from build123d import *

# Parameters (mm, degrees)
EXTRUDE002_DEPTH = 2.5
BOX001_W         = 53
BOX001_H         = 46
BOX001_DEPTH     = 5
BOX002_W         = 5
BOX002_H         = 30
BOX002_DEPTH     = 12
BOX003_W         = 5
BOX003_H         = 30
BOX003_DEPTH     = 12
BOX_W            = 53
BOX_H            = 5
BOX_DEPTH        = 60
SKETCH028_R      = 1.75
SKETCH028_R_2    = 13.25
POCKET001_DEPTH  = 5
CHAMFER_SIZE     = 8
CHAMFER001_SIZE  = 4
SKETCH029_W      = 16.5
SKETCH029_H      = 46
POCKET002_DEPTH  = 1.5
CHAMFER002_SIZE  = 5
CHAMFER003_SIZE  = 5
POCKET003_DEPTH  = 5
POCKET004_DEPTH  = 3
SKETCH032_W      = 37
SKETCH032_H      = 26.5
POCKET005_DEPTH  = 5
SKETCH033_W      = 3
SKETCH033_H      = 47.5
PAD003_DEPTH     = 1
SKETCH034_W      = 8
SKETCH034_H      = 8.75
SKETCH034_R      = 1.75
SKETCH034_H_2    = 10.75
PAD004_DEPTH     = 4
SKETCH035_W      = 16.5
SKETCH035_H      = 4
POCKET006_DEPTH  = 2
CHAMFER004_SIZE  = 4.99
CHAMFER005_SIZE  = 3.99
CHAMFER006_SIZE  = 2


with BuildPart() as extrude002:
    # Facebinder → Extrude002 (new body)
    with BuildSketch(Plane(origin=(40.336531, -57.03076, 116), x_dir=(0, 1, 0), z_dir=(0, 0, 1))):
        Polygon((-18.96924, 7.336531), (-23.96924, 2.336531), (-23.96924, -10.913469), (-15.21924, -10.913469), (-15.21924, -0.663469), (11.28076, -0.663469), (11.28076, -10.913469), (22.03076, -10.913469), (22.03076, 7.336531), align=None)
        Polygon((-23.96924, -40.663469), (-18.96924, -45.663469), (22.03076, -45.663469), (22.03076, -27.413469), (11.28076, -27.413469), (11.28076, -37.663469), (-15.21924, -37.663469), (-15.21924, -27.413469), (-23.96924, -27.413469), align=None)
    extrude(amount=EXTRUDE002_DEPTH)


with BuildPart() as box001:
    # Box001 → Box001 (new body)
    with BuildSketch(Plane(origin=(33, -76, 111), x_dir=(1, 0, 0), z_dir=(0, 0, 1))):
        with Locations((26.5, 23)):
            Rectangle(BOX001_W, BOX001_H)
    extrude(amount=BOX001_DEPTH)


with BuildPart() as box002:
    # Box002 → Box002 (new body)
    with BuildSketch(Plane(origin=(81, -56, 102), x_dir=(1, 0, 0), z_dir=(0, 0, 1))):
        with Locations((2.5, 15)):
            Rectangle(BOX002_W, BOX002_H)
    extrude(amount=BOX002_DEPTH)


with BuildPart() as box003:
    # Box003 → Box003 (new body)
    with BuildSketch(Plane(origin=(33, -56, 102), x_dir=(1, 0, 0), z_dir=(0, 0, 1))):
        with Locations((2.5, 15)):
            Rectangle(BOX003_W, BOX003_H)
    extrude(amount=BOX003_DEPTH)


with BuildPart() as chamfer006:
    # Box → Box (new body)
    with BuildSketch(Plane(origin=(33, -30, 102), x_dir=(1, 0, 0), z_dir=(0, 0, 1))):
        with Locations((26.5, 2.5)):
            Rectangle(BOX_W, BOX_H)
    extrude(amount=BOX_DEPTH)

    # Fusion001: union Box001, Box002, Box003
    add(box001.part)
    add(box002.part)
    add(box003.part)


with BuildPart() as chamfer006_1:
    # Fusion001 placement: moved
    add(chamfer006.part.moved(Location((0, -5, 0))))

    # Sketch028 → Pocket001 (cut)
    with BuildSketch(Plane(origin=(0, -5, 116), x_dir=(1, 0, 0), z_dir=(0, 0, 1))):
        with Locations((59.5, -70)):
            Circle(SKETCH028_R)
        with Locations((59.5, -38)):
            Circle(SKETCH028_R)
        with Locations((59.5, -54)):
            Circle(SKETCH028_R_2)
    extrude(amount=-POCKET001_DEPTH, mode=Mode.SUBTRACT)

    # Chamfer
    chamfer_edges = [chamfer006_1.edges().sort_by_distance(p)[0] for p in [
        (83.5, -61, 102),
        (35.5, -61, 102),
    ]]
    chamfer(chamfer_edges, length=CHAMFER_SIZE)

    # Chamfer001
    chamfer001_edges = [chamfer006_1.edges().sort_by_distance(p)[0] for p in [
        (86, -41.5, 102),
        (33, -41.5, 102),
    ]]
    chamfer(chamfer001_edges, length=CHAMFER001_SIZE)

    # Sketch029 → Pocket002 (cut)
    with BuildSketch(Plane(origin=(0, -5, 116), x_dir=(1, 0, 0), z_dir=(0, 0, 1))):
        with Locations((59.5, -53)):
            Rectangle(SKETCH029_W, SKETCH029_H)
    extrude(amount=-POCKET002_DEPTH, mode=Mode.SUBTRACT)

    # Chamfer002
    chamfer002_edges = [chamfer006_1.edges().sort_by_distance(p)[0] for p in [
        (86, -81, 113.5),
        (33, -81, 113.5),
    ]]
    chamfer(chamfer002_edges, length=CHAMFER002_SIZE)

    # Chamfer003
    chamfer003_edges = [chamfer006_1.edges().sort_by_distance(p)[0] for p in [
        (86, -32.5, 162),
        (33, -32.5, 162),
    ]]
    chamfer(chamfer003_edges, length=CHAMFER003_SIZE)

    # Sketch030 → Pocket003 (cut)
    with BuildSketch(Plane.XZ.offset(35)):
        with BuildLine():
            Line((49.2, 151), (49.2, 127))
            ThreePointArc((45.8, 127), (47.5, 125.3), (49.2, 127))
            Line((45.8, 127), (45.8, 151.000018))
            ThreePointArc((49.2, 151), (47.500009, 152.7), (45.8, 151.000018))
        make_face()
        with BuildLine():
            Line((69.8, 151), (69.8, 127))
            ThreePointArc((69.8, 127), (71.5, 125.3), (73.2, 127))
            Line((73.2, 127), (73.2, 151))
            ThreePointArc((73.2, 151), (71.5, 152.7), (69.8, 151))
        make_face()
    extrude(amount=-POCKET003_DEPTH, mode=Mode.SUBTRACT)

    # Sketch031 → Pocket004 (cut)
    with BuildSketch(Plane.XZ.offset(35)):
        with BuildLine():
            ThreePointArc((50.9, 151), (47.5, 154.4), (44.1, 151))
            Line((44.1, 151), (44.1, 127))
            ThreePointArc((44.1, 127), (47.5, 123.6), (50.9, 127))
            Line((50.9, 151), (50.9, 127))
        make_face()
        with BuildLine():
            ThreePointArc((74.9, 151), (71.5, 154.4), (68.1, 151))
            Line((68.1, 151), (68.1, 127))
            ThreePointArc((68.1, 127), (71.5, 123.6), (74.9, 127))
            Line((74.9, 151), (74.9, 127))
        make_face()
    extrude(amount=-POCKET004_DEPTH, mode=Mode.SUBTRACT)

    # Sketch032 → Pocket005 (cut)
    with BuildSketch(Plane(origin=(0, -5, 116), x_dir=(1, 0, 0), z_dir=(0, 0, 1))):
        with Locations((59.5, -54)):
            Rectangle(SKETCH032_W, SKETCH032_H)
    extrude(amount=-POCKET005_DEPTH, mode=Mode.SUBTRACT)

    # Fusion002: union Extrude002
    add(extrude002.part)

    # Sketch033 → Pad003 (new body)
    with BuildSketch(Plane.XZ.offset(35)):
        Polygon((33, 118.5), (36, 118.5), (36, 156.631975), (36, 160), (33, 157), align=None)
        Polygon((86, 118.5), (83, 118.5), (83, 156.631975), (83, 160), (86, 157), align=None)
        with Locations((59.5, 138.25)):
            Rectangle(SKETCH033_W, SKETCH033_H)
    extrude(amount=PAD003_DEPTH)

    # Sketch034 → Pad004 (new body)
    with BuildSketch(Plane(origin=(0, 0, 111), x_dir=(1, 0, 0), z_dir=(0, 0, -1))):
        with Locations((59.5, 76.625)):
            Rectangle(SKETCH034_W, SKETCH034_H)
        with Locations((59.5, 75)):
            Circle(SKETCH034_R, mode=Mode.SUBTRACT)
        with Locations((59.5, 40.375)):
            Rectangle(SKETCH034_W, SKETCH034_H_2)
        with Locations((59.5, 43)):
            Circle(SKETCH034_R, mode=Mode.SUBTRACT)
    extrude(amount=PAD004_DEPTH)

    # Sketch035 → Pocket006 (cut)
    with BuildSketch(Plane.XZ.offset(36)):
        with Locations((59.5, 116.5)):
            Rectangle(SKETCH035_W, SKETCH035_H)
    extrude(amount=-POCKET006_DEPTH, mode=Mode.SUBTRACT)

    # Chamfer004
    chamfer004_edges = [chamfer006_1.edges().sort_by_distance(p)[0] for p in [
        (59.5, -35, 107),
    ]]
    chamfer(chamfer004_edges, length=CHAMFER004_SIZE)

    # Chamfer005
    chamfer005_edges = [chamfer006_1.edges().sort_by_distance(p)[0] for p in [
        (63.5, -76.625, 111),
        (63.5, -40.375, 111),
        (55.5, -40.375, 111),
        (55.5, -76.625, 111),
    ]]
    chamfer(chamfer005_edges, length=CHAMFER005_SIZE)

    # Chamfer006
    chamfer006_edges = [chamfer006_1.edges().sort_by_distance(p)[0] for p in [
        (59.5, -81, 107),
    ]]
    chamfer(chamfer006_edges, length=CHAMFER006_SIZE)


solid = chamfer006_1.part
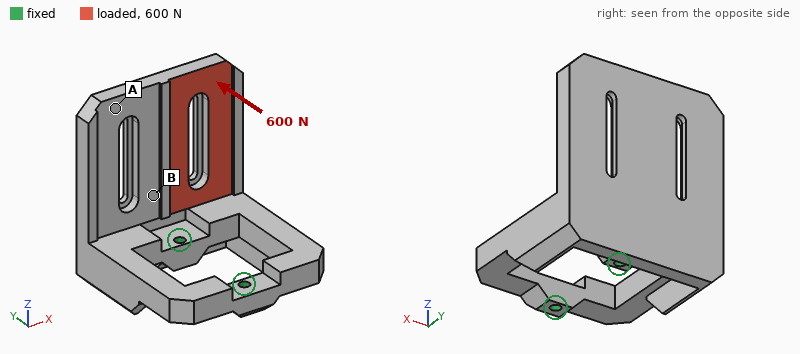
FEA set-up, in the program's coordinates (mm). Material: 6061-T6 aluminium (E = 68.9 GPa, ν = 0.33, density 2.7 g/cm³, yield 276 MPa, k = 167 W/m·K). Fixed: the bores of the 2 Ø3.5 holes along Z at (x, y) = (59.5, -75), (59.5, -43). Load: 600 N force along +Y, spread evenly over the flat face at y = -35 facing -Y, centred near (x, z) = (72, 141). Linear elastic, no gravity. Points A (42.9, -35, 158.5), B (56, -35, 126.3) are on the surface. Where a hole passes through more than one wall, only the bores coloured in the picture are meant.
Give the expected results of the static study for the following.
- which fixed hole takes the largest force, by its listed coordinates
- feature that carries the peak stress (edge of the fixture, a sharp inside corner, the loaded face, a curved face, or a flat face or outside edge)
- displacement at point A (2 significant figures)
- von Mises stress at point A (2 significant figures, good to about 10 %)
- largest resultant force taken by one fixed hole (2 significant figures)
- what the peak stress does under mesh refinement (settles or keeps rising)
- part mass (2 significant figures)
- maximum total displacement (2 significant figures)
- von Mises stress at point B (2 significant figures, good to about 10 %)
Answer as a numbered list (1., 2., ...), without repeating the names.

1. (59.5, -43)
2. edge of the fixture
3. 0.24 mm
4. 12 MPa
5. 520 N
6. keeps rising
7. 71 g
8. 0.40 mm
9. 40 MPa
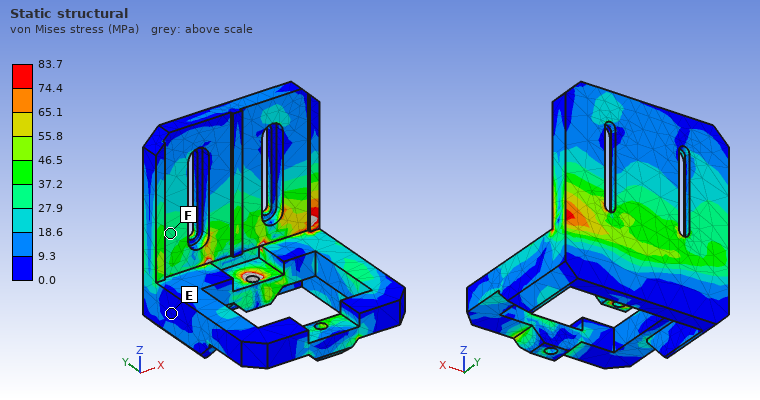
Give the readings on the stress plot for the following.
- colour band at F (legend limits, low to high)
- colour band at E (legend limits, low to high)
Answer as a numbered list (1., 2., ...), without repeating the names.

1. 27.9 to 37.2 MPa
2. 0.0 to 9.3 MPa
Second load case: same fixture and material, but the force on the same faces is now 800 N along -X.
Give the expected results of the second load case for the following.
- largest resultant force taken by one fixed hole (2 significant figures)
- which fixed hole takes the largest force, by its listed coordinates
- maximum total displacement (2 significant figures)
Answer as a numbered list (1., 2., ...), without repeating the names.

1. 890 N
2. (59.5, -43)
3. 0.25 mm
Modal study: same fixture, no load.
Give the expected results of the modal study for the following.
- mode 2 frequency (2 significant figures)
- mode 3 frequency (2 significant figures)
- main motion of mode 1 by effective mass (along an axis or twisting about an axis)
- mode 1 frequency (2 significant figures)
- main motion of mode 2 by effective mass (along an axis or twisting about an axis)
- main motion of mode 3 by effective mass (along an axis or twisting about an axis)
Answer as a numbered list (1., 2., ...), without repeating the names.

1. 1800 Hz
2. 3400 Hz
3. along Y
4. 1600 Hz
5. along X
6. twisting about Z
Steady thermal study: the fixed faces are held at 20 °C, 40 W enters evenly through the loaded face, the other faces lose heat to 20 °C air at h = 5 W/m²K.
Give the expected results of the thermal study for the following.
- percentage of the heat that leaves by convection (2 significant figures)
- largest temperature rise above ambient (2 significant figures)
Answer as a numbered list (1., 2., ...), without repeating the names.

1. 3.1 %
2. 52 K
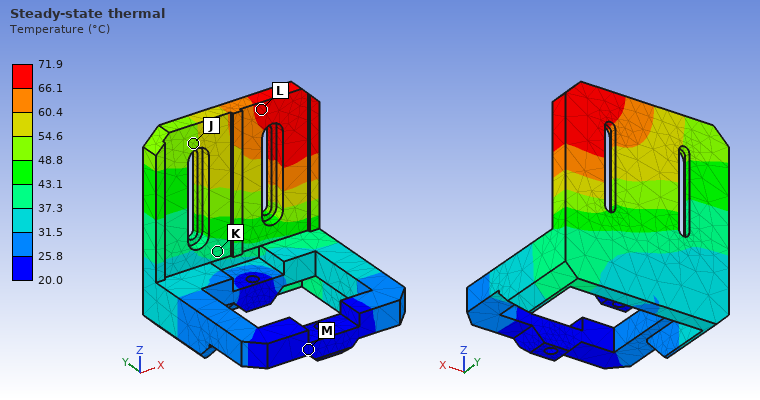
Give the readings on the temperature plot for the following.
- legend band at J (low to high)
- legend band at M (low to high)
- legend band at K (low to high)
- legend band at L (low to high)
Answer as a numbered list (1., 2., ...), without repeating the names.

1. 48.8 to 54.6 °C
2. 20.0 to 25.8 °C
3. 37.3 to 43.1 °C
4. 66.1 to 71.9 °C
